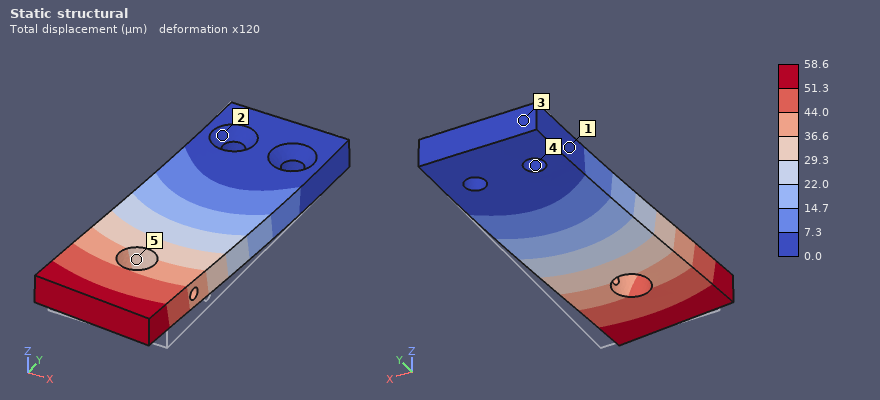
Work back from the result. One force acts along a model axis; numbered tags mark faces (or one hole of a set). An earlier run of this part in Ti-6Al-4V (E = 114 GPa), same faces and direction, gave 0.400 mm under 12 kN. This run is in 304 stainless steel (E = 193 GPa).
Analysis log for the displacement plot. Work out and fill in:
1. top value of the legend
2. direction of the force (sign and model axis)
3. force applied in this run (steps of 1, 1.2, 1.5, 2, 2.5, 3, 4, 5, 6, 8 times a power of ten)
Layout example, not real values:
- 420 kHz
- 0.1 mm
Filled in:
- 58.6 µm
- -X
- 3 kN
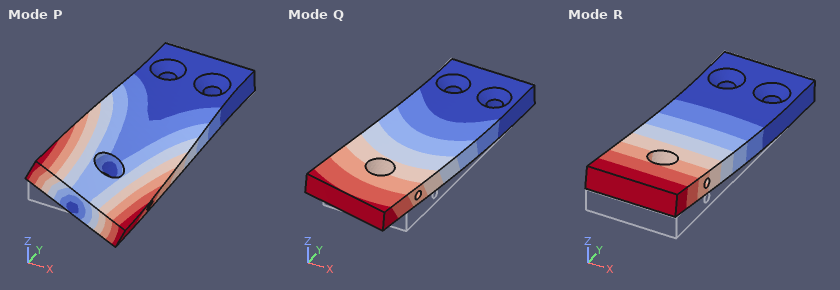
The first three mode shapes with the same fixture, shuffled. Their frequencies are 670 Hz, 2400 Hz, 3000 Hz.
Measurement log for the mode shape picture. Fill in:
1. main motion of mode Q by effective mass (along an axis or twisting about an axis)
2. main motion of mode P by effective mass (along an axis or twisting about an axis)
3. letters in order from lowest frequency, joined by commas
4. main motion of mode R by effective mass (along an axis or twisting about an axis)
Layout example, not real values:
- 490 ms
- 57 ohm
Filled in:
- along X
- twisting about Y
- R, Q, P
- along Z
